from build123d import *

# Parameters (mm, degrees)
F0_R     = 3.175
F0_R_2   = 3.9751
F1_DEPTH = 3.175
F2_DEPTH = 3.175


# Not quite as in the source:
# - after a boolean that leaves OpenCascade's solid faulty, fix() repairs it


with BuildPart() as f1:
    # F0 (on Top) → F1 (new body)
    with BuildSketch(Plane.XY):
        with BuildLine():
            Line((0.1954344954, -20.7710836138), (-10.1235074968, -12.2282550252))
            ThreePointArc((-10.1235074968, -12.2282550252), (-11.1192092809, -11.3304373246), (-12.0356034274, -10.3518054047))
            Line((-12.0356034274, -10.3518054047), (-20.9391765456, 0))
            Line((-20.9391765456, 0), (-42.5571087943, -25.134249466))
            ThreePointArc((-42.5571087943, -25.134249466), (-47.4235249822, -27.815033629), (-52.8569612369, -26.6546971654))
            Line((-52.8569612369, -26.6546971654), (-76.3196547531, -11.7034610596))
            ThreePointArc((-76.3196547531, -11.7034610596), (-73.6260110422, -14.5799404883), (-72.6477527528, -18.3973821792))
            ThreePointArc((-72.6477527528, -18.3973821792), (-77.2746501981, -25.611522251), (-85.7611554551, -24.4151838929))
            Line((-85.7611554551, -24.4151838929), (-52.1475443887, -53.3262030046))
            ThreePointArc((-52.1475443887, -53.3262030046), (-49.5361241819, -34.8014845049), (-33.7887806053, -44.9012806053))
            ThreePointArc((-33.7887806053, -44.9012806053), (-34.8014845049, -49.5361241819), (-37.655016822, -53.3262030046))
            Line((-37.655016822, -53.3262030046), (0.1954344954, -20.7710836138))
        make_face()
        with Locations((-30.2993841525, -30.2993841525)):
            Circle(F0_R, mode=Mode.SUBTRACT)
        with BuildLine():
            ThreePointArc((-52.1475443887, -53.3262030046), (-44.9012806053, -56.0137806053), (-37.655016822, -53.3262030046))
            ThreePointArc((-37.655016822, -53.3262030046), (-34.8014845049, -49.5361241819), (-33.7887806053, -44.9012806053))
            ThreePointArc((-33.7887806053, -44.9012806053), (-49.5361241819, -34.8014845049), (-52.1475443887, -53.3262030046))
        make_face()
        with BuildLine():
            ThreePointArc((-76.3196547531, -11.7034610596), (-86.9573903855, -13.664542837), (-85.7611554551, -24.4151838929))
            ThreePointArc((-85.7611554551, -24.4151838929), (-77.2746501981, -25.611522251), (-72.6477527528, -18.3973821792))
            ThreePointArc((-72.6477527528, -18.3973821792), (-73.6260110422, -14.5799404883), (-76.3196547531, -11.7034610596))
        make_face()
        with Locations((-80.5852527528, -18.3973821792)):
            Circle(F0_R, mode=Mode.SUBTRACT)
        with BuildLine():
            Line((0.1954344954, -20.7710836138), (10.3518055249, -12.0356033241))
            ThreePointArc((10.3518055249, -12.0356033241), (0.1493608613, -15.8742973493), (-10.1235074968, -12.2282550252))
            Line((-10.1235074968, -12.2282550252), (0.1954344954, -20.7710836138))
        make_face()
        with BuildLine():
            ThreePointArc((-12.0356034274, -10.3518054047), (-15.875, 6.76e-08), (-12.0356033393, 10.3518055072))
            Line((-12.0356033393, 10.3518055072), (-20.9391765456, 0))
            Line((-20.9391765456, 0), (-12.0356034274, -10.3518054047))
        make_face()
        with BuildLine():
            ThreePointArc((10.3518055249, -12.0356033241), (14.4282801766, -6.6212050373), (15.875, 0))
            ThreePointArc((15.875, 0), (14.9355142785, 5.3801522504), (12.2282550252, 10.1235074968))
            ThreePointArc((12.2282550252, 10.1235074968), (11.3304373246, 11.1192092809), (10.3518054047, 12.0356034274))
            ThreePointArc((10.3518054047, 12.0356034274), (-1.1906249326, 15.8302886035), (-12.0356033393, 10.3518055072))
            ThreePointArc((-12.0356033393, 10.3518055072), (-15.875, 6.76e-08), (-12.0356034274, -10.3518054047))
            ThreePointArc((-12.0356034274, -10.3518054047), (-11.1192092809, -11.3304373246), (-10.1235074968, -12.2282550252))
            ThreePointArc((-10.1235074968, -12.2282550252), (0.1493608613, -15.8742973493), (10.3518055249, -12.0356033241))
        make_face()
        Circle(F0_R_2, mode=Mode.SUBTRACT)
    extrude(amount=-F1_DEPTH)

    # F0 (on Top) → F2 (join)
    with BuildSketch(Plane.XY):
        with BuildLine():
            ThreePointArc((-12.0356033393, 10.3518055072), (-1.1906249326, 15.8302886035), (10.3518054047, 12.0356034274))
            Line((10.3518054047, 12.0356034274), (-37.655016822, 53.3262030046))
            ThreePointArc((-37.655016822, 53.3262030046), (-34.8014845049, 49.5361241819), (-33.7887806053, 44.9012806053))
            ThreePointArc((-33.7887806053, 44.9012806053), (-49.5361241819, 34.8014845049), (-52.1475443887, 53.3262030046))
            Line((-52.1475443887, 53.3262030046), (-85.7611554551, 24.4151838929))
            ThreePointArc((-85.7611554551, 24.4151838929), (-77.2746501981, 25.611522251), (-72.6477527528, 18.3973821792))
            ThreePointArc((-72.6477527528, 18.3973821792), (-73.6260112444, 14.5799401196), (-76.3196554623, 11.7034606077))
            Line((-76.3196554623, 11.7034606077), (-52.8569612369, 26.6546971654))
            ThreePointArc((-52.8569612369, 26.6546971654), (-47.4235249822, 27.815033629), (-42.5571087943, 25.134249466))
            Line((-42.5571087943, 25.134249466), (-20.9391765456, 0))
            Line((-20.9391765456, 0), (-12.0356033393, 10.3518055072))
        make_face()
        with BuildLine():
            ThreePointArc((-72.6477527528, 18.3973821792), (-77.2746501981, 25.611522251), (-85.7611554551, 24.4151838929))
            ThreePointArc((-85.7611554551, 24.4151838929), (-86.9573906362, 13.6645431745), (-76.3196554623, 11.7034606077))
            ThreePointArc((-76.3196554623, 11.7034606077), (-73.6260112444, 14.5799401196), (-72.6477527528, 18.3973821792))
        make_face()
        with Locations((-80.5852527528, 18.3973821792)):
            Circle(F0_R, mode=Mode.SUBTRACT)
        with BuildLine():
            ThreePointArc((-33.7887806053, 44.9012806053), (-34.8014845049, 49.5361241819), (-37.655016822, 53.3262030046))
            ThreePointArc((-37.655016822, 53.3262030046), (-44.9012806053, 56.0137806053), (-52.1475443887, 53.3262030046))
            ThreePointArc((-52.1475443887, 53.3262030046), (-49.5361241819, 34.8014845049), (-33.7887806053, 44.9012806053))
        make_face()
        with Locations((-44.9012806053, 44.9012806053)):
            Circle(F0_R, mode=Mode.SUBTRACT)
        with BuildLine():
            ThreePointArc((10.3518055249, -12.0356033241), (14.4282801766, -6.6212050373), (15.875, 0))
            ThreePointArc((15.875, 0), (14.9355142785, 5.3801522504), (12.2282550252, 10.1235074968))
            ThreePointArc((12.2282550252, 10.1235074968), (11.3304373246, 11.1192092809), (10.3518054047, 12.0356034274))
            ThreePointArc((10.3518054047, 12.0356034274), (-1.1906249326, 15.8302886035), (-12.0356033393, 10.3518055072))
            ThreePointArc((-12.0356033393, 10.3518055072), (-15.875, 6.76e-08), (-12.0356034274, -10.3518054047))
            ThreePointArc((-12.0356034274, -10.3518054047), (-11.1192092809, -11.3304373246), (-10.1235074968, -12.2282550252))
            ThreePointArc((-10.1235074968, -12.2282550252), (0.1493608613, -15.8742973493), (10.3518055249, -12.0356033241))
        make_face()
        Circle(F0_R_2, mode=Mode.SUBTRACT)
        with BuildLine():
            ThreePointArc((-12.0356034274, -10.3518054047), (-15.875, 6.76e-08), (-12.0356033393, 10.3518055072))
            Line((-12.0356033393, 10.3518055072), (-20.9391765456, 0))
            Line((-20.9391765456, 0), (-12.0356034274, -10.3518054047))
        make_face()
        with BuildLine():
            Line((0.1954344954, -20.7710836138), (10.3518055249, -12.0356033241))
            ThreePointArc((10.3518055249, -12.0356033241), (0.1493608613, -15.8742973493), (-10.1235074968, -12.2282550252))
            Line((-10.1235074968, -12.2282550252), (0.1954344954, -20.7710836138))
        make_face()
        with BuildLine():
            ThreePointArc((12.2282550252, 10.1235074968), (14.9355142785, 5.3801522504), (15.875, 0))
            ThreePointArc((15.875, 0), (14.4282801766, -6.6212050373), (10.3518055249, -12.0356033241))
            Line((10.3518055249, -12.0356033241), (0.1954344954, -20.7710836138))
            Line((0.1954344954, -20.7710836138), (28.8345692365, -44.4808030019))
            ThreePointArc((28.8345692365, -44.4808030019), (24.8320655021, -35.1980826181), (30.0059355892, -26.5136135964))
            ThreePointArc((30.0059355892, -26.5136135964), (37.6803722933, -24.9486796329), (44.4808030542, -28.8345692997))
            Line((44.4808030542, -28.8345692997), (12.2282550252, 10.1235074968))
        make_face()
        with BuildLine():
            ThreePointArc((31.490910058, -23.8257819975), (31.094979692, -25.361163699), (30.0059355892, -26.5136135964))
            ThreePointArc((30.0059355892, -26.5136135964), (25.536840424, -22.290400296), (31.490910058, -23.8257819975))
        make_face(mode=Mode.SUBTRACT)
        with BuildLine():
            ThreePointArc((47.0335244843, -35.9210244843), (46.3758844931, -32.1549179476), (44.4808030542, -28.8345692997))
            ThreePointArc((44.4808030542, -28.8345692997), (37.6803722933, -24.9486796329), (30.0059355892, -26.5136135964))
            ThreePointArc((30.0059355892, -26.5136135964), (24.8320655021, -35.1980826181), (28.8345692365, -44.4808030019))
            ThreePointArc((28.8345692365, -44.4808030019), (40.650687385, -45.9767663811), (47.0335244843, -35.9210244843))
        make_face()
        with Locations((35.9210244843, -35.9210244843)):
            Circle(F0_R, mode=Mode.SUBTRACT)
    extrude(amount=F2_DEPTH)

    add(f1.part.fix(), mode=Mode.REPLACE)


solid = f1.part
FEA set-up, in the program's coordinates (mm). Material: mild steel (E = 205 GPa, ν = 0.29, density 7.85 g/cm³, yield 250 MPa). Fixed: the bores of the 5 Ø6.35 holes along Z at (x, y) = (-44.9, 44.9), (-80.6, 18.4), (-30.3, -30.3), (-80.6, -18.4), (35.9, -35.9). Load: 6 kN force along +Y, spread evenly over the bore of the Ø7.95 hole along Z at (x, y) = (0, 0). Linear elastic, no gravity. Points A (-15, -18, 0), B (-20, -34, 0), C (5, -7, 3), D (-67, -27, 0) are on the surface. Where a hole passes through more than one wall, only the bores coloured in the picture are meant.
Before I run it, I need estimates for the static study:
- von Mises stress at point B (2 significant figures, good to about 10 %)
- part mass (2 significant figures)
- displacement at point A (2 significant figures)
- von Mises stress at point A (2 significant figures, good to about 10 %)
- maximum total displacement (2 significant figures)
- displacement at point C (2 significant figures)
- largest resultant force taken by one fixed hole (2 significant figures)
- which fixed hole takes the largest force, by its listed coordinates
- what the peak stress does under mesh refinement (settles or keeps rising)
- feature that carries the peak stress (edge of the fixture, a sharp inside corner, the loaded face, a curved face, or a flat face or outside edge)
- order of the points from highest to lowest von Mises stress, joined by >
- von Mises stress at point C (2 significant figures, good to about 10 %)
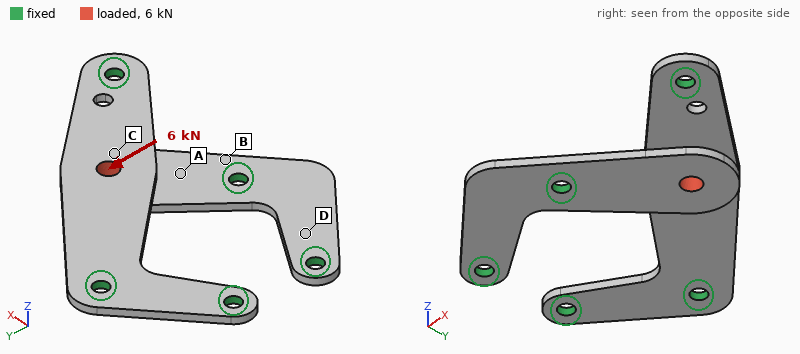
37 MPa
170 g
6.5 µm
65 MPa
36 µm
23 µm
3.5 kN
(-30.3, -30.3)
keeps rising
edge of the fixture
A > B > C > D
24 MPa
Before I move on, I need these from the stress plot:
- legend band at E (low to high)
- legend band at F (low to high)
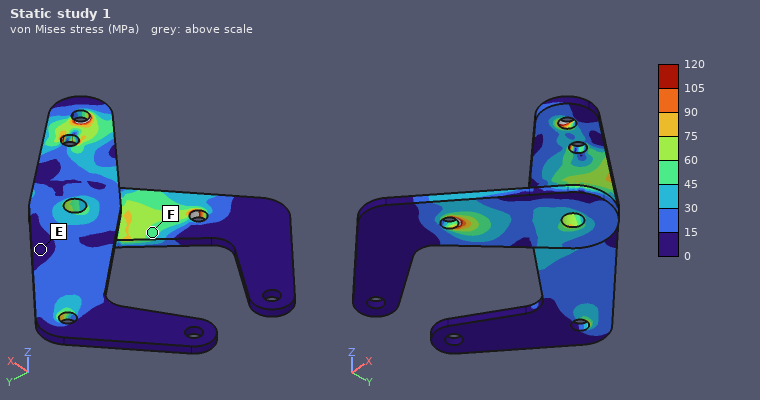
0 to 15 MPa
45 to 60 MPa
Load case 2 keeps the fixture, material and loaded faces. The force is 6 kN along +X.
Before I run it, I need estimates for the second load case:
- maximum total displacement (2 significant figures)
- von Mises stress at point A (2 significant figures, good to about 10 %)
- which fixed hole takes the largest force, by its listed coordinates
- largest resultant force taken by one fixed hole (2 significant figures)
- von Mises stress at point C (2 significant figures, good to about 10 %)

55 µm
65 MPa
(-30.3, -30.3)
3.4 kN
35 MPa
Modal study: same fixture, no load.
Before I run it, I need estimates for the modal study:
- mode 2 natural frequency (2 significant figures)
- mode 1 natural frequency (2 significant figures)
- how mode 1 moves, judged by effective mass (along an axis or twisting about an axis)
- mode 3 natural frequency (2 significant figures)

3700 Hz
1600 Hz
along Z
3900 Hz
